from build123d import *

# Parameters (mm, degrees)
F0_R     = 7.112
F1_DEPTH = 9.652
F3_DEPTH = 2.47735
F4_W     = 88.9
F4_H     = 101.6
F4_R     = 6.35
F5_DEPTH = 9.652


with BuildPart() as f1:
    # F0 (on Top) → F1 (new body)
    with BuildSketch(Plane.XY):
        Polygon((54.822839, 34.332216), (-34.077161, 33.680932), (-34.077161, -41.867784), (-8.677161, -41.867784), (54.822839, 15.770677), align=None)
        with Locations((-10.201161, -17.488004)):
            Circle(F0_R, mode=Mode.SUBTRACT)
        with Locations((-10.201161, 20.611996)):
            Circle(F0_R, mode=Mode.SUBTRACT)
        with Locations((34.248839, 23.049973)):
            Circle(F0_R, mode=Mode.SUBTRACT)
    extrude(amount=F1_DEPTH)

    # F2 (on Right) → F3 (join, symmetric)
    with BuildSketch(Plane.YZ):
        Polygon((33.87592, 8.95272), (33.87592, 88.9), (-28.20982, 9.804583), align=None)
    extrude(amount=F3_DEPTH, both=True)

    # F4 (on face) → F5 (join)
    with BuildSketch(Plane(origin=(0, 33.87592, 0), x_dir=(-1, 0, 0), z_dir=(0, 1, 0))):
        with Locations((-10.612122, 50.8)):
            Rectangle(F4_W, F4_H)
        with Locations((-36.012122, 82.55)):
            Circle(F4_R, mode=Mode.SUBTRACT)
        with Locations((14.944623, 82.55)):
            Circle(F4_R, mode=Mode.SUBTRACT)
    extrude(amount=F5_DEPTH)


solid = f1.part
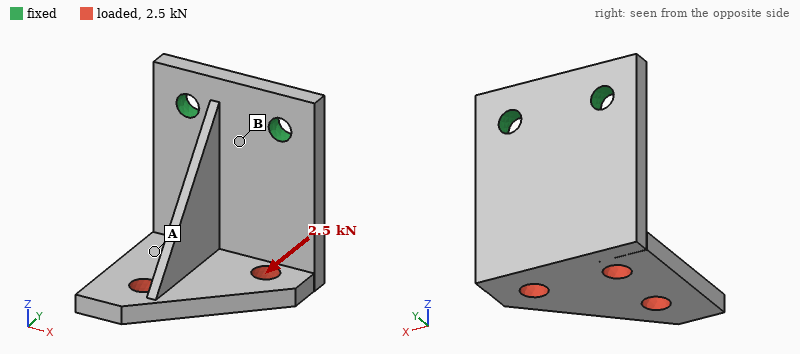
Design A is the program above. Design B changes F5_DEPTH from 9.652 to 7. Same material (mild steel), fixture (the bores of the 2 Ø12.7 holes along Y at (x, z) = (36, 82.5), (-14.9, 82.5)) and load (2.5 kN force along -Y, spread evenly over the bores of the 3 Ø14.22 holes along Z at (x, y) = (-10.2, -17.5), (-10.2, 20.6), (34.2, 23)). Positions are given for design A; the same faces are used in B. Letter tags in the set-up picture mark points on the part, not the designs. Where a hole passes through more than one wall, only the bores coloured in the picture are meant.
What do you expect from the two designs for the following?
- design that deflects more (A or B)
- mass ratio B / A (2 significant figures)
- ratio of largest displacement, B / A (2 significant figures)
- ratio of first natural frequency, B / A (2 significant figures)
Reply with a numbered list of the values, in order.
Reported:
1. B
2. 0.83
3. 2.0
4. 0.74
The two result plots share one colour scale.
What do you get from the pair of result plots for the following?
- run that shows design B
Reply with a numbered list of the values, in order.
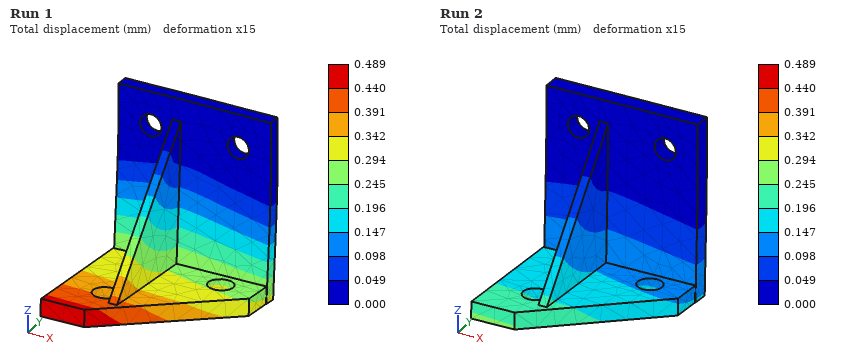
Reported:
1. Run 1
